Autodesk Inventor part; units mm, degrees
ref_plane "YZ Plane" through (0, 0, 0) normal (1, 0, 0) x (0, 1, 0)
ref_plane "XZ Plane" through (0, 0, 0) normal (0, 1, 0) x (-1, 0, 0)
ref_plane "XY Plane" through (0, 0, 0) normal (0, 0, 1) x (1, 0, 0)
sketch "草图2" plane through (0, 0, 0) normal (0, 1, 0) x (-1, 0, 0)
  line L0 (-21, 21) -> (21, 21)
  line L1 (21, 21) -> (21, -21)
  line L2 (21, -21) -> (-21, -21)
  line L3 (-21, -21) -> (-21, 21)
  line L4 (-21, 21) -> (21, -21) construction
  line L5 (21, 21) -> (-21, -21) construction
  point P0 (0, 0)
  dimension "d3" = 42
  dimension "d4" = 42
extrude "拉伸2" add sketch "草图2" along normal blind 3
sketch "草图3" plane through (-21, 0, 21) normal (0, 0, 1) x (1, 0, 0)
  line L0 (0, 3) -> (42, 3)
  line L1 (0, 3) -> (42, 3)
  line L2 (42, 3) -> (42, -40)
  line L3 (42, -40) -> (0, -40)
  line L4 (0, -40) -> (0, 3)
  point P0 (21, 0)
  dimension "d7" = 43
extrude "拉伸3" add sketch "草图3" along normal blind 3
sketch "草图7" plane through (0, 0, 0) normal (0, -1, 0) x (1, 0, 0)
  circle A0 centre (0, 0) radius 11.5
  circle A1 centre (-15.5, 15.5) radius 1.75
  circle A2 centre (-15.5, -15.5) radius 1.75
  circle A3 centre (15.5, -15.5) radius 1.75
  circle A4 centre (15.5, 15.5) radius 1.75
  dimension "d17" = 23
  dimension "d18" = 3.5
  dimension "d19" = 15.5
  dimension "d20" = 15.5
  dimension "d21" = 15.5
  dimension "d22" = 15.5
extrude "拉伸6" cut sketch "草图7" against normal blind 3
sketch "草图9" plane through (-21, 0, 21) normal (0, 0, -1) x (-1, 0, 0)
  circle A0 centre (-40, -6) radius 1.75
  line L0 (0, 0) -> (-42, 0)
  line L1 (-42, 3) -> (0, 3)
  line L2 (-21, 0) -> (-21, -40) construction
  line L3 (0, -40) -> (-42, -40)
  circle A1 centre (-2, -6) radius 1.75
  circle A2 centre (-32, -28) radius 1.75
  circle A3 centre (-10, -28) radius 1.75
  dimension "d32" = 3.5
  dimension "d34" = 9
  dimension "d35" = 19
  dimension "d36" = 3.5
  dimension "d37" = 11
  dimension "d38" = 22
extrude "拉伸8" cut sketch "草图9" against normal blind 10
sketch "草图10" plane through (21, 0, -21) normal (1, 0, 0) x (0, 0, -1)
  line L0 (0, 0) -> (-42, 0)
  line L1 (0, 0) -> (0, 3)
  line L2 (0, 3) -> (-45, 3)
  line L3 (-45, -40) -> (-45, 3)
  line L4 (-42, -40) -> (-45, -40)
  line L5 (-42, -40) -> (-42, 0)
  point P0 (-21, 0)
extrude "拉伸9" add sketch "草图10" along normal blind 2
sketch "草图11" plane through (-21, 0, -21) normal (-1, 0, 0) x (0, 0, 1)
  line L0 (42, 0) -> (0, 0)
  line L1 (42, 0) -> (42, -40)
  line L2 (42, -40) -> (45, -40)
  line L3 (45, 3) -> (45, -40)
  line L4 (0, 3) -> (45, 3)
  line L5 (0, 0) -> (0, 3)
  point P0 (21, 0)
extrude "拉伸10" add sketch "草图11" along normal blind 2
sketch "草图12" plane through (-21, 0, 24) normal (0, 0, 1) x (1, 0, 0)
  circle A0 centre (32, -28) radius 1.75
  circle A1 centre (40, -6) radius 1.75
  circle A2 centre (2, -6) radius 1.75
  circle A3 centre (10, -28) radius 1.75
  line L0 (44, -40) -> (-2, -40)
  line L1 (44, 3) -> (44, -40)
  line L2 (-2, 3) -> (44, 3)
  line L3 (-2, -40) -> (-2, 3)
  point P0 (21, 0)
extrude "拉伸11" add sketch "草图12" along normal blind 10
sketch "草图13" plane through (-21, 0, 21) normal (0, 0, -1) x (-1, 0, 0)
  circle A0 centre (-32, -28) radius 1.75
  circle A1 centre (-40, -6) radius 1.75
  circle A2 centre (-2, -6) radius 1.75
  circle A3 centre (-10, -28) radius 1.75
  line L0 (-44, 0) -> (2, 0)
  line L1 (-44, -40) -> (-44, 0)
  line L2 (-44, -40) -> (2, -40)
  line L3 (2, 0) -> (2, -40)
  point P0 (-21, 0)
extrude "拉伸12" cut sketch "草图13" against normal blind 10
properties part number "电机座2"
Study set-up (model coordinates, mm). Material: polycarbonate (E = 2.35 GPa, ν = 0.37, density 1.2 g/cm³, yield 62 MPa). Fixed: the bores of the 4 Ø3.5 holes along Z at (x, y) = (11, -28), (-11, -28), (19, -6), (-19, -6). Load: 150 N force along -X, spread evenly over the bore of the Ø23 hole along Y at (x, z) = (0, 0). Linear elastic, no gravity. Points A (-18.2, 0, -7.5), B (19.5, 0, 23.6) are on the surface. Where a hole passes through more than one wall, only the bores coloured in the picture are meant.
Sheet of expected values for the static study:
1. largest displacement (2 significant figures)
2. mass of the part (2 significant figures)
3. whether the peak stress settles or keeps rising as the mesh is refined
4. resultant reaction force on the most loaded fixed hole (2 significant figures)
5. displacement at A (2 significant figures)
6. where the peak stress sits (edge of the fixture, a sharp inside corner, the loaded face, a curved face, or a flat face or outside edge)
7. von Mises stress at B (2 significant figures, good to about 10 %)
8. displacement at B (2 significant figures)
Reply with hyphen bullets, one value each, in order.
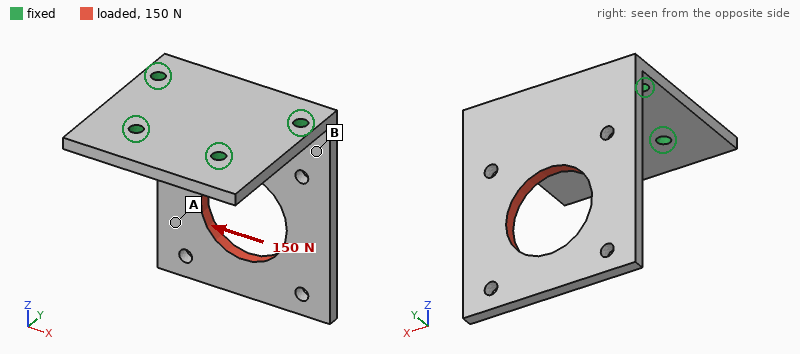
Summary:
- 0.86 mm
- 14 g
- keeps rising
- 150 N
- 0.66 mm
- edge of the fixture
- 8.2 MPa
- 0.27 mm
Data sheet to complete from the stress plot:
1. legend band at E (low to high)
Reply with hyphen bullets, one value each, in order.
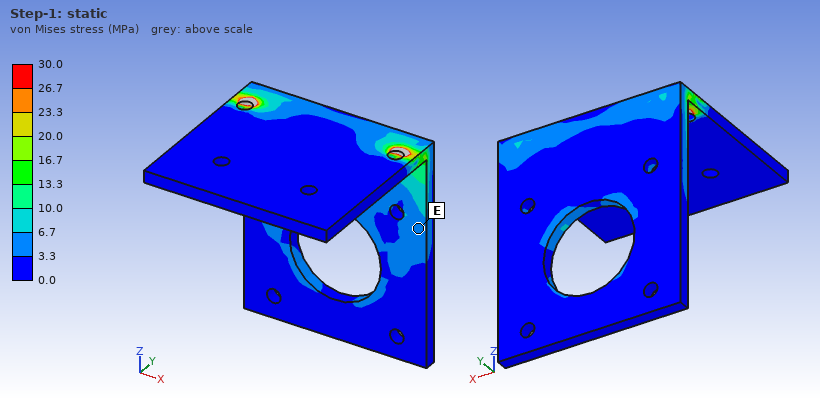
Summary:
- 3.3 to 6.7 MPa
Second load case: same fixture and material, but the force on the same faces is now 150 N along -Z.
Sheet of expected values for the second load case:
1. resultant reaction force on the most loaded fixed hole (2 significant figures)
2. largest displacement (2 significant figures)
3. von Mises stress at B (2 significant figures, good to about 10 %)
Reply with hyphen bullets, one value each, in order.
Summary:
- 82 N
- 0.99 mm
- 2.7 MPa
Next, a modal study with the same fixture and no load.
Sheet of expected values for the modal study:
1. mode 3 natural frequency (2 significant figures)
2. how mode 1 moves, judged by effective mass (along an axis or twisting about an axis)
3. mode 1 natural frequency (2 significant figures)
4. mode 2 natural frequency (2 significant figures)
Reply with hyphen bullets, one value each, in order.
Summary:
- 1100 Hz
- along Y
- 210 Hz
- 540 Hz
